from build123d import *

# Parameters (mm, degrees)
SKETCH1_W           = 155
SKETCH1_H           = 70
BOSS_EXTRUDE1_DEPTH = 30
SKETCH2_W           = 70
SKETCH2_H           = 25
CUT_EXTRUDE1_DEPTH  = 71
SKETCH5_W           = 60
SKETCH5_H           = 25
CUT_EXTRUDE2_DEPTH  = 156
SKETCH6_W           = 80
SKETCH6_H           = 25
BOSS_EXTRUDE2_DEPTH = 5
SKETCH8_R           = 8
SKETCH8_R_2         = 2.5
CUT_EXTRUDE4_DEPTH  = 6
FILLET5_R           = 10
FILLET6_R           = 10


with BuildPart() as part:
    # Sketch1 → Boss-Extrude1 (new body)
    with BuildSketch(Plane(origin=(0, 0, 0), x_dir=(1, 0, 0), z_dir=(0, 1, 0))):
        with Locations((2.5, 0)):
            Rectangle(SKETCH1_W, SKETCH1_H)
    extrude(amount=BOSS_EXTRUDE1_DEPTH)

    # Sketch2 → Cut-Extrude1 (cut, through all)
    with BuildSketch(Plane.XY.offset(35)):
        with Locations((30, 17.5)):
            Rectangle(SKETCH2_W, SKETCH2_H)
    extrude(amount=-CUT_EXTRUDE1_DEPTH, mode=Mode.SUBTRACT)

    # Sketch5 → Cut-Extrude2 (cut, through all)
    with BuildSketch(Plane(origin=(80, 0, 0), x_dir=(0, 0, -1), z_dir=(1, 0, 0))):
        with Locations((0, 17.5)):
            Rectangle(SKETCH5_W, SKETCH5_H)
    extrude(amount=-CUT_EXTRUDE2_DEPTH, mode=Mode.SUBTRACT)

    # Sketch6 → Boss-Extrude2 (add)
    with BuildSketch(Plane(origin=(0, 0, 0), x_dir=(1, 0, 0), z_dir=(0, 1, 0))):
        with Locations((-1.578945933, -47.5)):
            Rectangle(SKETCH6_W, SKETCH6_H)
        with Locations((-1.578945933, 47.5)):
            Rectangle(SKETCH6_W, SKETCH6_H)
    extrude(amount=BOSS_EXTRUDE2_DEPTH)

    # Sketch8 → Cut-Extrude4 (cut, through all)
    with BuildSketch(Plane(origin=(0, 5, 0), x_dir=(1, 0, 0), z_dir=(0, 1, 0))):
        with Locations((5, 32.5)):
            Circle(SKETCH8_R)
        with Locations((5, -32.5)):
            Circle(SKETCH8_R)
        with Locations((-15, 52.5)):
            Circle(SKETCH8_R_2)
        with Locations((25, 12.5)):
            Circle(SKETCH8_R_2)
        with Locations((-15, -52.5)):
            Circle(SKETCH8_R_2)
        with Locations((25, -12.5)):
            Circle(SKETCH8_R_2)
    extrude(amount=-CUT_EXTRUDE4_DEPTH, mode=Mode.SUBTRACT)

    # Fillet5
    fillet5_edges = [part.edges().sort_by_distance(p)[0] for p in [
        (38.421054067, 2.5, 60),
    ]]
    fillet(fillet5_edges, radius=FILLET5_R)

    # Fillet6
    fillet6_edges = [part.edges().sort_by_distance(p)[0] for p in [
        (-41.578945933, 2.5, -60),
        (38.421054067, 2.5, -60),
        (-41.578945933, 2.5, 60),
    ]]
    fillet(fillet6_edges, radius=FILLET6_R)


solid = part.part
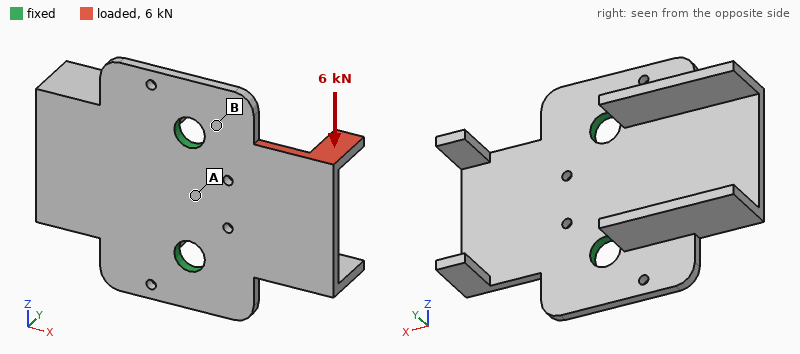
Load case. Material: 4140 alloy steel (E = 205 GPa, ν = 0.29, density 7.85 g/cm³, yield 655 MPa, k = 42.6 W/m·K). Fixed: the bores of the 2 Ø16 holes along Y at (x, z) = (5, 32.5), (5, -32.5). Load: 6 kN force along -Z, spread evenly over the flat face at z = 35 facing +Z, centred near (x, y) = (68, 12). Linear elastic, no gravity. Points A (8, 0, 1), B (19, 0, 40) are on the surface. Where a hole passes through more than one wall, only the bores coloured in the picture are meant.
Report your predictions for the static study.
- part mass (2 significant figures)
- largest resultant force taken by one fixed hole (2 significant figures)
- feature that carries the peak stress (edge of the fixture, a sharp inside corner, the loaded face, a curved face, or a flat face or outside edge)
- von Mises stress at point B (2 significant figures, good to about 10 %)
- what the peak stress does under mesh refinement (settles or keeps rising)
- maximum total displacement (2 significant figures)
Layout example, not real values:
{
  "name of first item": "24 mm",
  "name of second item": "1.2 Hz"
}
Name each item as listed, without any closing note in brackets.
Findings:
{
  "part mass": "730 g",
  "largest resultant force taken by one fixed hole": "5.9 kN",
  "feature that carries the peak stress": "a sharp inside corner",
  "von Mises stress at point B": "120 MPa",
  "what the peak stress does under mesh refinement": "keeps rising",
  "maximum total displacement": "1.1 mm"
}
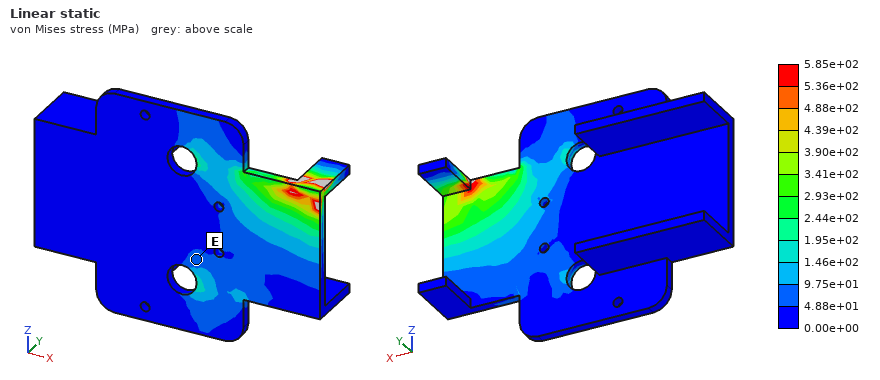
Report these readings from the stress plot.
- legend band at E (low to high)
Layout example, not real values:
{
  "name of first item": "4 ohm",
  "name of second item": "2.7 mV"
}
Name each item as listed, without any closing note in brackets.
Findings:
{
  "legend band at E": "4.88e+01 to 9.75e+01 MPa"
}
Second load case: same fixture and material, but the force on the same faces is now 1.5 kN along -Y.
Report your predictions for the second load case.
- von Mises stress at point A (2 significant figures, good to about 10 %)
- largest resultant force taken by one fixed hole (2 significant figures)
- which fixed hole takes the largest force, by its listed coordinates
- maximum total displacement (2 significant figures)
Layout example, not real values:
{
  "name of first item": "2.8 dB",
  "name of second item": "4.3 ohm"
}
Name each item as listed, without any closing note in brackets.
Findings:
{
  "von Mises stress at point A": "79 MPa",
  "largest resultant force taken by one fixed hole": "1.5 kN",
  "which fixed hole takes the largest force, by its listed coordinates": "(5, 32.5)",
  "maximum total displacement": "1.1 mm"
}
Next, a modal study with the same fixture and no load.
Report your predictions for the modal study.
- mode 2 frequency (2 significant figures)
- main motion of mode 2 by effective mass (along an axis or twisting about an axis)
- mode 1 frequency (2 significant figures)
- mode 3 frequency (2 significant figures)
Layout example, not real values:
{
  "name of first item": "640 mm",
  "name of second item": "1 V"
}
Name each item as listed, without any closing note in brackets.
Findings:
{
  "mode 2 frequency": "880 Hz",
  "main motion of mode 2 by effective mass": "along Y",
  "mode 1 frequency": "760 Hz",
  "mode 3 frequency": "1500 Hz"
}
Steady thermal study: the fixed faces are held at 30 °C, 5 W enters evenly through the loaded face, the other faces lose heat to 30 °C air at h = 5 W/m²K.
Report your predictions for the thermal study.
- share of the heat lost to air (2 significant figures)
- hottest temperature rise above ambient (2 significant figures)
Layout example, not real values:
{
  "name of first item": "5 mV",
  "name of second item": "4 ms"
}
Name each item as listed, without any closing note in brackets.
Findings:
{
  "share of the heat lost to air": "15 %",
  "hottest temperature rise above ambient": "42 K"
}
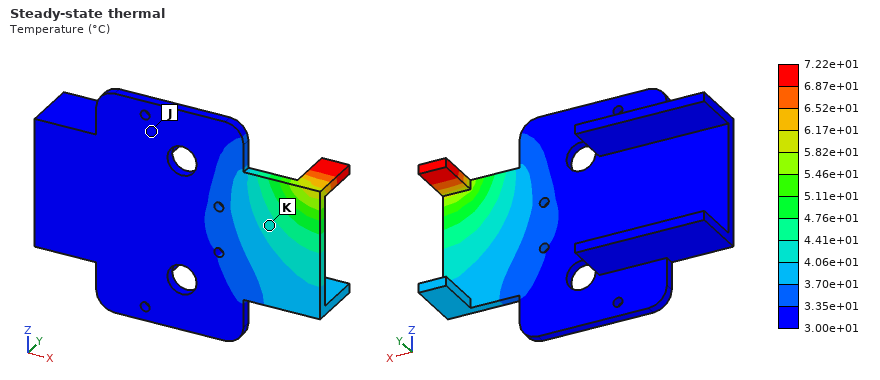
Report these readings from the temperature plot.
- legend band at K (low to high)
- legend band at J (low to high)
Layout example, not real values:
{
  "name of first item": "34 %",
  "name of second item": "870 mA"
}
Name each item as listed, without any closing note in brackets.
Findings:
{
  "legend band at K": "4.06e+01 to 4.41e+01 °C",
  "legend band at J": "3.00e+01 to 3.35e+01 °C"
}
